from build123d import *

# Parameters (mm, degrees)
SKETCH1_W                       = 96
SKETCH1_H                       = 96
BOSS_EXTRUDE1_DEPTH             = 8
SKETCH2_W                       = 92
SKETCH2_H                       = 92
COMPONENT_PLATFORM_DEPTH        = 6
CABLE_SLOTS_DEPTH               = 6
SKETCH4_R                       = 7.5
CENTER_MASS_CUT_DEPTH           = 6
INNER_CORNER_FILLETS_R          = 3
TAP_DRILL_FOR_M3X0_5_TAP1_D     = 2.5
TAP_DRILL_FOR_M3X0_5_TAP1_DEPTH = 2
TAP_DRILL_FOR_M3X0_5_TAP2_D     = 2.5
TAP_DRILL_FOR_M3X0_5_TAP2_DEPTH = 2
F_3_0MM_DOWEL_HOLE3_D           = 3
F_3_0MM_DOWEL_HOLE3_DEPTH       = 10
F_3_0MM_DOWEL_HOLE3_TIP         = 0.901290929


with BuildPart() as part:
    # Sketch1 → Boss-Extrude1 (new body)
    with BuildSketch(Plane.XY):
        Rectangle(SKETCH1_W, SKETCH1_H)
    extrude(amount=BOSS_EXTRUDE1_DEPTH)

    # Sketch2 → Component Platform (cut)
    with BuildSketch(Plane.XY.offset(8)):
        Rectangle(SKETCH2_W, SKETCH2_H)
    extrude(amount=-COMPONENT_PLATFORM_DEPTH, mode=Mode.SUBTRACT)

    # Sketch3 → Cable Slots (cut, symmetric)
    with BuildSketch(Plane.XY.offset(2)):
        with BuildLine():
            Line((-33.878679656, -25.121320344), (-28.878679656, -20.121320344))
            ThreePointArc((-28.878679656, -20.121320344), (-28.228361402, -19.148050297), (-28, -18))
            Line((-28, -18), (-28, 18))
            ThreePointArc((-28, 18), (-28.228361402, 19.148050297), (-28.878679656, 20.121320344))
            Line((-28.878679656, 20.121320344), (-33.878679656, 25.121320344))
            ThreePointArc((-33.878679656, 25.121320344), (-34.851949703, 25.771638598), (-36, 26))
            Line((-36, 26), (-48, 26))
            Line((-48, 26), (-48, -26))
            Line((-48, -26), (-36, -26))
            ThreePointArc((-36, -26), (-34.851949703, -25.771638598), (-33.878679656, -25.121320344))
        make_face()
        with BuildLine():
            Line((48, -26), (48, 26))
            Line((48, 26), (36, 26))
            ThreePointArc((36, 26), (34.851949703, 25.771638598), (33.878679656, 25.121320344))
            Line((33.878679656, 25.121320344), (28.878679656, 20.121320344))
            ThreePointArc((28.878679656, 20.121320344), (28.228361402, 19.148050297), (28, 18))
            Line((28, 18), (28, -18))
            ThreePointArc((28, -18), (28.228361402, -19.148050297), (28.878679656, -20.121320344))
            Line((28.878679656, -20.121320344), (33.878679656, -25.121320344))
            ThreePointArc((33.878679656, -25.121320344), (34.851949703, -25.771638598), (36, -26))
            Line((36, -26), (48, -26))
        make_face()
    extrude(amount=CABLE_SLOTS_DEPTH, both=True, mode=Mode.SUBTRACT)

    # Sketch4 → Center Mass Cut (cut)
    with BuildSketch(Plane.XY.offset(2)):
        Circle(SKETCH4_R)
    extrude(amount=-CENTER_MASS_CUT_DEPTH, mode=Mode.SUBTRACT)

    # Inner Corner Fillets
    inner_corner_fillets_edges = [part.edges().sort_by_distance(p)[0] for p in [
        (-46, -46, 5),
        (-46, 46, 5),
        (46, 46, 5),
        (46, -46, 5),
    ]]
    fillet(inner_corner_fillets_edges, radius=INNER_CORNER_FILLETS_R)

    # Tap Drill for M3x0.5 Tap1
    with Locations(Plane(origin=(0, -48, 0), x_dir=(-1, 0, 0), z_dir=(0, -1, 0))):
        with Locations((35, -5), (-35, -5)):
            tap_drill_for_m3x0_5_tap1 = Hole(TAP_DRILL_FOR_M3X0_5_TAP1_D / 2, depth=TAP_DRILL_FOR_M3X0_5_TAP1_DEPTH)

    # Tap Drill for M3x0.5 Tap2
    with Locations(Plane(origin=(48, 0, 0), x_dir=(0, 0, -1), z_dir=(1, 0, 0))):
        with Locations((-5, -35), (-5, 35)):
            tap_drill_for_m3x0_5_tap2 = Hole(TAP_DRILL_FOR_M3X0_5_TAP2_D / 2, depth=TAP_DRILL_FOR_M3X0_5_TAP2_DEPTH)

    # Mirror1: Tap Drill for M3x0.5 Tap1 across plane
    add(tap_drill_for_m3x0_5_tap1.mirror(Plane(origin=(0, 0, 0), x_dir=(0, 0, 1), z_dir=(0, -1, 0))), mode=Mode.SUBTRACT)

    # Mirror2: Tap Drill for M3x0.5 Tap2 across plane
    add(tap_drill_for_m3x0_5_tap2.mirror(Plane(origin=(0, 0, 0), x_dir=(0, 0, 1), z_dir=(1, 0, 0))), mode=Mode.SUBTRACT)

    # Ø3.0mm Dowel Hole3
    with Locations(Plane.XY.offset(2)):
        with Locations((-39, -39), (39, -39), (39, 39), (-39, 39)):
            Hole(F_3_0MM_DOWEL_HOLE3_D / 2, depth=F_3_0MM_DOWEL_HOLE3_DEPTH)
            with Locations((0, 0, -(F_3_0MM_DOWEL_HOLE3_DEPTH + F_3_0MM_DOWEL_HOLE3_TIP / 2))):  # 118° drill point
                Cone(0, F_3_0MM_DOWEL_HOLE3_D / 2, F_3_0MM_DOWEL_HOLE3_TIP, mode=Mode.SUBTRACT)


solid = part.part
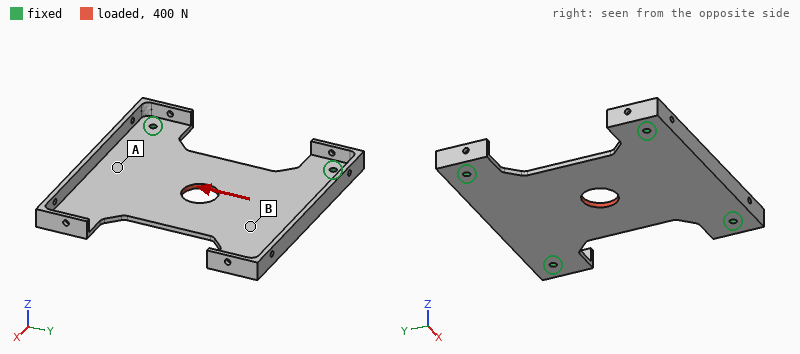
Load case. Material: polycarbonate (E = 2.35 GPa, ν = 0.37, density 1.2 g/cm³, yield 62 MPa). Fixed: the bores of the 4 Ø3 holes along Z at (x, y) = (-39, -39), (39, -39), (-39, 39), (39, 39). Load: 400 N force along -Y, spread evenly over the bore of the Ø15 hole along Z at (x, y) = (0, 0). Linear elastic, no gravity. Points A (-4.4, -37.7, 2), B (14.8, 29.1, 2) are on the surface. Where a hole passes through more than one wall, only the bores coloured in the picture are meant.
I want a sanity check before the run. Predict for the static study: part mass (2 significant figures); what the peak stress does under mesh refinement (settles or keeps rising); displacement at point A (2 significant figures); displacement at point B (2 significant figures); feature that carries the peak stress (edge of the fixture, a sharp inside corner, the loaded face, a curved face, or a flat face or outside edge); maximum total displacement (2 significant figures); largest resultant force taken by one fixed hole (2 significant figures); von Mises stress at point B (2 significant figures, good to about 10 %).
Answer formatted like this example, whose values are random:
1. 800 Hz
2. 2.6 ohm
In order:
1. 21 g
2. keeps rising
3. 0.11 mm
4. 0.092 mm
5. edge of the fixture
6. 0.15 mm
7. 110 N
8. 2.1 MPa
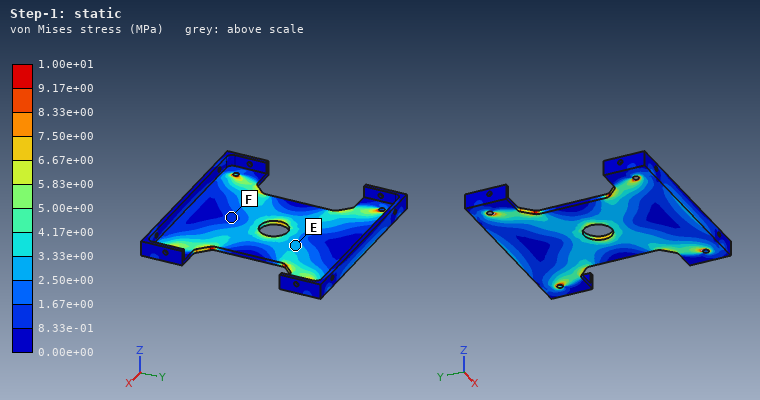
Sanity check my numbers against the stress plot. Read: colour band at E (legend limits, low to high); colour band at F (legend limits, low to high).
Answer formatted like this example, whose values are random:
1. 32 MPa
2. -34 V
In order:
1. 2.50e+00 to 3.33e+00 MPa
2. 8.33e-01 to 1.67e+00 MPa
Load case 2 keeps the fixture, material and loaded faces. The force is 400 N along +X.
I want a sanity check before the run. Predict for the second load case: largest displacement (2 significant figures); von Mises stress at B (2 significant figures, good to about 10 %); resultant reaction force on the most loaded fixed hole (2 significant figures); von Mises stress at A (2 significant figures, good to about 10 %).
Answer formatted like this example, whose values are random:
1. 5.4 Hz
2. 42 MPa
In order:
1. 0.10 mm
2. 2.2 MPa
3. 120 N
4. 0.85 MPa
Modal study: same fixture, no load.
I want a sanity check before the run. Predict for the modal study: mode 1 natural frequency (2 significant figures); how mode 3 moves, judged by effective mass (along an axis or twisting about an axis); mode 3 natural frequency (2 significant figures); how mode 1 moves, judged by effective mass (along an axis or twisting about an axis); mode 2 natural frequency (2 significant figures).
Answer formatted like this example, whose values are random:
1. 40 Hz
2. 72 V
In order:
1. 330 Hz
2. twisting about X
3. 730 Hz
4. along Z
5. 660 Hz
